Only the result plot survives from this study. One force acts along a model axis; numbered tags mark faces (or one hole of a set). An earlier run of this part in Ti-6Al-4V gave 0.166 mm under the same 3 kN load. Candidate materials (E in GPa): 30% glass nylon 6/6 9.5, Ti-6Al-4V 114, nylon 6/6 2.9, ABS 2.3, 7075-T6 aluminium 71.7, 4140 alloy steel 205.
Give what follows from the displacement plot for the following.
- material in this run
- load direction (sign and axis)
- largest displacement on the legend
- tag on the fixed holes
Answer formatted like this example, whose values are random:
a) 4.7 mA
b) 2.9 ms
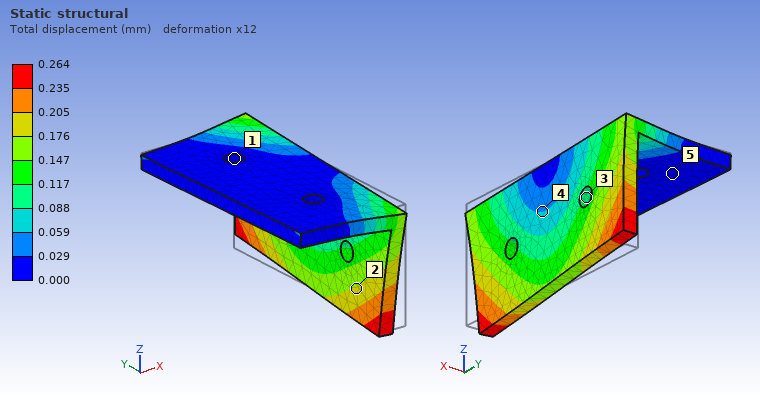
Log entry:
a) 7075-T6 aluminium
b) +Y
c) 0.264 mm
d) 1
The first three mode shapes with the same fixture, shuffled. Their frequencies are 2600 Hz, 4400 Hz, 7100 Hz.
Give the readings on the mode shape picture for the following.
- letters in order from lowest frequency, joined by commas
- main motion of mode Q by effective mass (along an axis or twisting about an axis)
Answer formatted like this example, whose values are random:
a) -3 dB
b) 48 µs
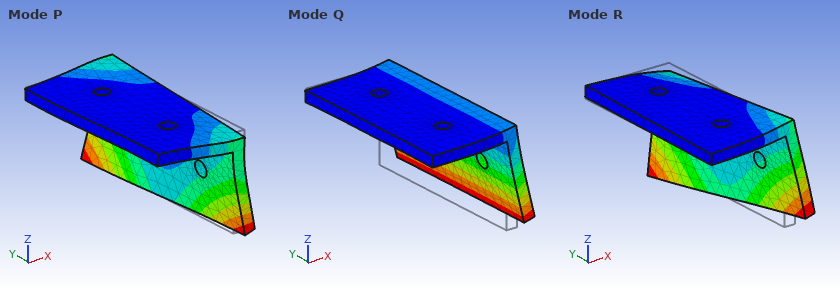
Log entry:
a) Q, R, P
b) along X
